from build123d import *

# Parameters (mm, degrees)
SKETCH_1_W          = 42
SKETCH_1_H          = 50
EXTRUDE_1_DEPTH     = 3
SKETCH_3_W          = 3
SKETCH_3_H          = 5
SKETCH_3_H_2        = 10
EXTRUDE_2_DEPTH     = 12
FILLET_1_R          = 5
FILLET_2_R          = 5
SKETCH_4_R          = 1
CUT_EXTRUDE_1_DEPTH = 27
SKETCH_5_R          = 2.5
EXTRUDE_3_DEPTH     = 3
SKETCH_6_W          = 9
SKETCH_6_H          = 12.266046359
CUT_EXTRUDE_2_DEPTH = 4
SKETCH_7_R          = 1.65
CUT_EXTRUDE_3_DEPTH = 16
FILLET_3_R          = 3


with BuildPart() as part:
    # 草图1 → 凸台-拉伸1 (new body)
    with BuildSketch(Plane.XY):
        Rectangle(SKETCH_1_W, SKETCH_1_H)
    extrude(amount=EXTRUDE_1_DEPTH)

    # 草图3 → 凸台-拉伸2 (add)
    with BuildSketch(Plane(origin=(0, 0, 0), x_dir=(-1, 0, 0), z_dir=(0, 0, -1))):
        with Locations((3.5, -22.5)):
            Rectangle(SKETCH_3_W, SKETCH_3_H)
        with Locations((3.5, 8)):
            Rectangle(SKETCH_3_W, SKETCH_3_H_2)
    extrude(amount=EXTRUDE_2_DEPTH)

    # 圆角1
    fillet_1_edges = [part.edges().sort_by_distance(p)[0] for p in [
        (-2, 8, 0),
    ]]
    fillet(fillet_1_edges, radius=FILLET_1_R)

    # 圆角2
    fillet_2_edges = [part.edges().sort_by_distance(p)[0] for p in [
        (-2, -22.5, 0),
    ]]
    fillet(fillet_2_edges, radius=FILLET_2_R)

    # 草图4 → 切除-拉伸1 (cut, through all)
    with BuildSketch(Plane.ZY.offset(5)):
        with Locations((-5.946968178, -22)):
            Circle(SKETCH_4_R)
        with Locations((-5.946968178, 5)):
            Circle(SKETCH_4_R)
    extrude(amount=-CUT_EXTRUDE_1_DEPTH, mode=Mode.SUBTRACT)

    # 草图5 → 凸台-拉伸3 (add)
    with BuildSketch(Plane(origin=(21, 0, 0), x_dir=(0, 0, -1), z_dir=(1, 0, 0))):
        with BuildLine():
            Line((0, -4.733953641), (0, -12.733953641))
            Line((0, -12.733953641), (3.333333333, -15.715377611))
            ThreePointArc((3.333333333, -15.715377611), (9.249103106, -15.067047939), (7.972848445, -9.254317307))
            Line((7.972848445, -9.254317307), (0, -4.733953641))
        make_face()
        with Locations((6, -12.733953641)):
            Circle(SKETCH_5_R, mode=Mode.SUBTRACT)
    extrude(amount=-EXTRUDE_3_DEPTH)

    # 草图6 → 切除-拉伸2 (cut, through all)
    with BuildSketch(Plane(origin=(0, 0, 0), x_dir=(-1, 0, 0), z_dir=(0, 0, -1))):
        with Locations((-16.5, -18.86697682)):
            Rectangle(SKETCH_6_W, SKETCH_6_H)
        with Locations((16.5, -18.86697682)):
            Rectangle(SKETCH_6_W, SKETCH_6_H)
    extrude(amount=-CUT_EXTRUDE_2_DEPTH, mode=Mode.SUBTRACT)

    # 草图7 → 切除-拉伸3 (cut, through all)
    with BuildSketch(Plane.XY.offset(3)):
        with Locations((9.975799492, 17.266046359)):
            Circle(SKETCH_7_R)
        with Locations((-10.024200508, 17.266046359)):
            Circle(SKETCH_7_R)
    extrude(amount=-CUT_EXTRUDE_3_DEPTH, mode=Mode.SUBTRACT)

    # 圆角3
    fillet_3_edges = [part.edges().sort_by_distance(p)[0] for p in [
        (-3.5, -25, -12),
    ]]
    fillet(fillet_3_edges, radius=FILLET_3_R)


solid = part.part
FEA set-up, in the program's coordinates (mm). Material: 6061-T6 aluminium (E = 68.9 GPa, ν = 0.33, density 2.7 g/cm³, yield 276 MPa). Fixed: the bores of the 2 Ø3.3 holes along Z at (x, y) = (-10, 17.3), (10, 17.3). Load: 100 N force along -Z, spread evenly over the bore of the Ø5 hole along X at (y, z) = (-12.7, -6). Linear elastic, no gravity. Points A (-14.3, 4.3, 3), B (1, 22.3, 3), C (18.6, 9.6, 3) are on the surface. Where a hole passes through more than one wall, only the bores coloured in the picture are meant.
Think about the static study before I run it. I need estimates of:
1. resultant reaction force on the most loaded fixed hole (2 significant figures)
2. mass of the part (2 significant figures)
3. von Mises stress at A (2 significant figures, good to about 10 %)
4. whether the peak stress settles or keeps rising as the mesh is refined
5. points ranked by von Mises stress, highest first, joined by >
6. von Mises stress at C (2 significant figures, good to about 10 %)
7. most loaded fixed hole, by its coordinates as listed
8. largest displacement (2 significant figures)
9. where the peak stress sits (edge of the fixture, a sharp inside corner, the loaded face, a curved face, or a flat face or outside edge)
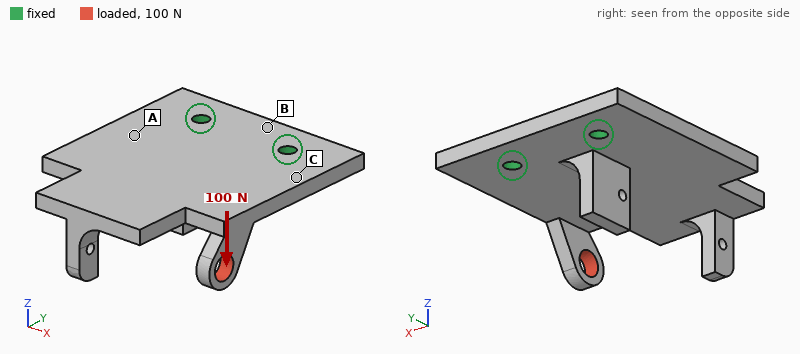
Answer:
130 N
17 g
20 MPa
keeps rising
C > A > B
46 MPa
(10, 17.3)
0.28 mm
edge of the fixture
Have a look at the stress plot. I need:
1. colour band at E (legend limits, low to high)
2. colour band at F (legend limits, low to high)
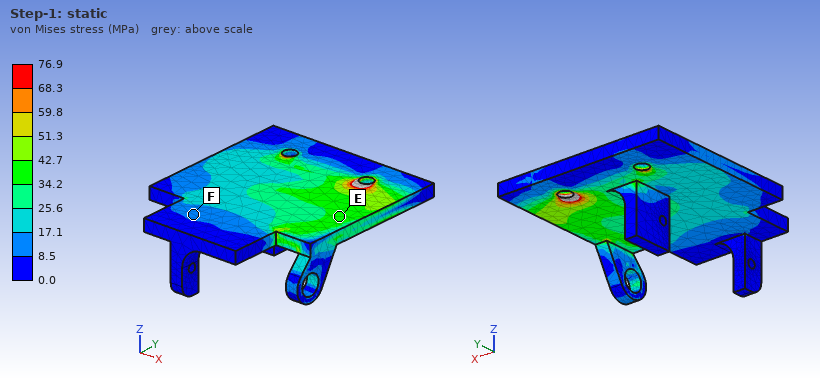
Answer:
34.2 to 42.7 MPa
8.5 to 17.1 MPa
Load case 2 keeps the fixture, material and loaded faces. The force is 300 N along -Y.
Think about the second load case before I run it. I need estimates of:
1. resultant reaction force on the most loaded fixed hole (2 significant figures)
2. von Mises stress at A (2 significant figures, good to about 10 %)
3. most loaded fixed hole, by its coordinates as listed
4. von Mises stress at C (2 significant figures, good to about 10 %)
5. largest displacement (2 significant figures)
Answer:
420 N
23 MPa
(10, 17.3)
35 MPa
0.33 mm
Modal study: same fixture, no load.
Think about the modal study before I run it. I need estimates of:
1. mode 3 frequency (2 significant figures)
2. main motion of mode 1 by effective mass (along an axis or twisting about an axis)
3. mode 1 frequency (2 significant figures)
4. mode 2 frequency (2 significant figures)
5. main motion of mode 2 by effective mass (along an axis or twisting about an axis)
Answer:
6500 Hz
along Z
1500 Hz
3800 Hz
twisting about Y
